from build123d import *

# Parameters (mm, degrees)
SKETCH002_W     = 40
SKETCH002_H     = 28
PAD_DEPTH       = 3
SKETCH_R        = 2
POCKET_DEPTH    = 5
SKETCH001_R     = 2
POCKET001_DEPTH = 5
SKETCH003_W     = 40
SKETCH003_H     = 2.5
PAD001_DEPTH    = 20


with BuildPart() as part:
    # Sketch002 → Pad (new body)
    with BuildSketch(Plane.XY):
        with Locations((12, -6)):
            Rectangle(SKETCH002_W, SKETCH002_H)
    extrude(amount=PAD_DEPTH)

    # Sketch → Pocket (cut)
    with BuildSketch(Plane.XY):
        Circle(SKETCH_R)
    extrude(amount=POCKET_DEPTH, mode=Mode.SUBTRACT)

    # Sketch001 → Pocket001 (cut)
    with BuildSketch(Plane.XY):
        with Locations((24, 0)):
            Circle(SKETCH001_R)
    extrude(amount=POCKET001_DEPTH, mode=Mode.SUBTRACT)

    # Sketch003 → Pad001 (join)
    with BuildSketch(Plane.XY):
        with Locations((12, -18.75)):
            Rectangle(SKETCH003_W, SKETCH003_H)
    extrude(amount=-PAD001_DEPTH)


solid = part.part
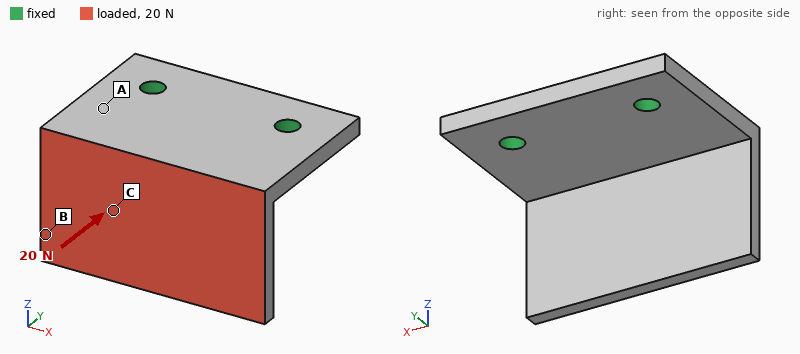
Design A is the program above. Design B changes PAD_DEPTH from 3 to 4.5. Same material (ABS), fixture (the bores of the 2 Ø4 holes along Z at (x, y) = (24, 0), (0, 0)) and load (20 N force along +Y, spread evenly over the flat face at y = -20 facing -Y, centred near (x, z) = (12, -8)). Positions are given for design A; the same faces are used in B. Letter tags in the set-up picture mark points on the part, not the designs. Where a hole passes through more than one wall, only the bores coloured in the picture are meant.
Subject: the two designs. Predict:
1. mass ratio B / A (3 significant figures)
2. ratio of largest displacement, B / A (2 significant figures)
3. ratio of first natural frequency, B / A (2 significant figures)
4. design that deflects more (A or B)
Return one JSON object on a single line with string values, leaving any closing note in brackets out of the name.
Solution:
{"mass ratio B / A": "1.31", "ratio of largest displacement, B / A": "0.51", "ratio of first natural frequency, B / A": "1.5", "design that deflects more": "A"}
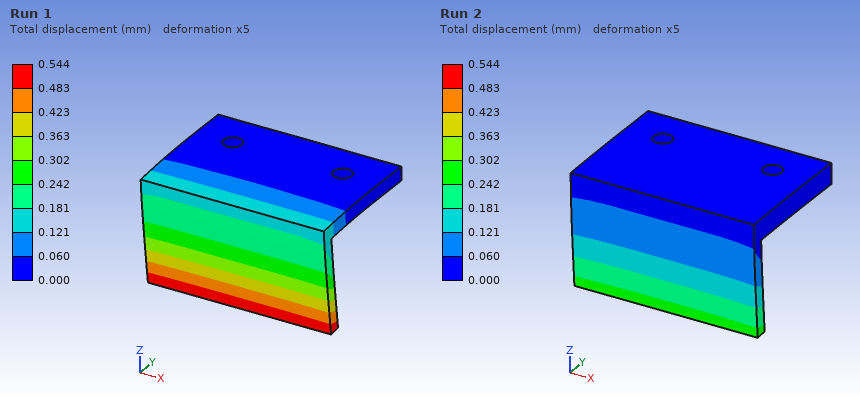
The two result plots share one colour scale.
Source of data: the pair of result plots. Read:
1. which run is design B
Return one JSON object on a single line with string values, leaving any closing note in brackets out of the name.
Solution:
{"which run is design B": "Run 2"}
